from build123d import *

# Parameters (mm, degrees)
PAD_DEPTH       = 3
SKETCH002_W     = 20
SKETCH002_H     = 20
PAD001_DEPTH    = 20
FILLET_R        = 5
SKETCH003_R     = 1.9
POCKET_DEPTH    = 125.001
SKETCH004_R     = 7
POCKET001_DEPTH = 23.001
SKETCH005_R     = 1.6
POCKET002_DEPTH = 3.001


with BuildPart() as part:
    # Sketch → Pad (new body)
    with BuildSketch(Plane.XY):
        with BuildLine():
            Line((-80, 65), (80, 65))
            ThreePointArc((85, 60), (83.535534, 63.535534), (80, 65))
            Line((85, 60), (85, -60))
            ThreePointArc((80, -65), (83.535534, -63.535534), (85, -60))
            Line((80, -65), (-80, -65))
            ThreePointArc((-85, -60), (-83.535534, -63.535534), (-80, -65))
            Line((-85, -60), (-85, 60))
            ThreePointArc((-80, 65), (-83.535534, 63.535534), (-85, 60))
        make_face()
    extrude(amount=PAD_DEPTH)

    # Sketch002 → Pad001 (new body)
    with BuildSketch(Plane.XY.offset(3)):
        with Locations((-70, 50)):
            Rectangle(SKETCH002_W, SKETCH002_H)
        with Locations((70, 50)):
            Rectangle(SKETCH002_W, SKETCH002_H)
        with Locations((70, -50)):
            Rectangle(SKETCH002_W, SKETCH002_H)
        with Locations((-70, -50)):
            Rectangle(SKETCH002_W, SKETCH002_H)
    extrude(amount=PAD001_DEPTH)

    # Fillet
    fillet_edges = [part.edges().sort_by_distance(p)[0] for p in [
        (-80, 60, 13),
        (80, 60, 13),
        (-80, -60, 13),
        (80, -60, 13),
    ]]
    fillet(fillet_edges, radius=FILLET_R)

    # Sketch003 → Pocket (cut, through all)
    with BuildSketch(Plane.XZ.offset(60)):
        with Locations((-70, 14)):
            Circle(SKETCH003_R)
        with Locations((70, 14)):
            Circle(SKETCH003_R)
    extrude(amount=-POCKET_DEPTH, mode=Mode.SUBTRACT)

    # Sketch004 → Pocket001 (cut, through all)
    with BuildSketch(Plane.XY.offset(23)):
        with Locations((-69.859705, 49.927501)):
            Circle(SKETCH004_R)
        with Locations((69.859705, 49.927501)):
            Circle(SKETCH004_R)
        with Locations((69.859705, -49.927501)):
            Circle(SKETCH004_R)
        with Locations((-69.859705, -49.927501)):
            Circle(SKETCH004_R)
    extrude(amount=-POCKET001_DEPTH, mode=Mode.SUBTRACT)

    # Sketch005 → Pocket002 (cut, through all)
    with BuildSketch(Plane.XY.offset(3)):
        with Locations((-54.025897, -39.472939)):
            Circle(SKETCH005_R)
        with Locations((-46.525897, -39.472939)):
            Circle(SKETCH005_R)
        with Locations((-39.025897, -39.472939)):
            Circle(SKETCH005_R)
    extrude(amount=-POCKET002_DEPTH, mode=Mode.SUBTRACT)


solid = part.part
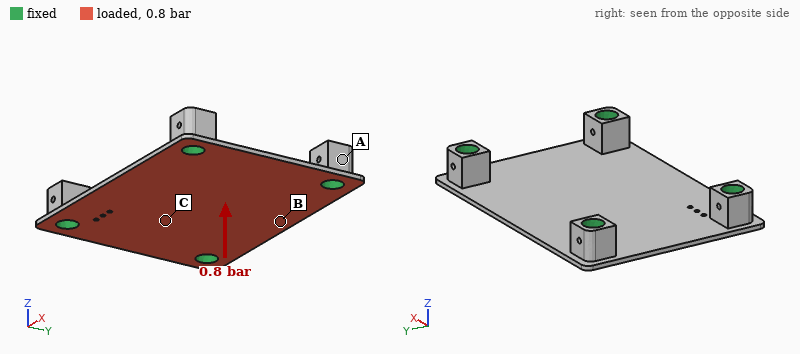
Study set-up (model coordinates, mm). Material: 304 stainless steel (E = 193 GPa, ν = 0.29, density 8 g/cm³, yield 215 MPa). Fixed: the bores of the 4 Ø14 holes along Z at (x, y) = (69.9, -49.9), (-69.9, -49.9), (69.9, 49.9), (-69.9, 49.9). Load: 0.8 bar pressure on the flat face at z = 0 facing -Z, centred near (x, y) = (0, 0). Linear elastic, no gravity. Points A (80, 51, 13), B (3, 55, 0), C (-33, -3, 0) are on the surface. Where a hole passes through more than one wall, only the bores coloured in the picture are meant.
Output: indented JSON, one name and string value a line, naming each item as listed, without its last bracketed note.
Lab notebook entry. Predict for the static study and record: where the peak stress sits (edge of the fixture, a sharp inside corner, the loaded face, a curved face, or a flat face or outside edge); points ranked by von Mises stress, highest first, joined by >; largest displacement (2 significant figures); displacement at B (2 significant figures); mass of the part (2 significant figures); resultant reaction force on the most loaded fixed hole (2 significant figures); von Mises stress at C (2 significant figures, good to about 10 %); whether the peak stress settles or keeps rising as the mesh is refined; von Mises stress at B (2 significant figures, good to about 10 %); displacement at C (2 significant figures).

{
  "where the peak stress sits": "a sharp inside corner",
  "points ranked by von Mises stress, highest first, joined by >": "B > C > A",
  "largest displacement": "0.17 mm",
  "displacement at B": "0.13 mm",
  "mass of the part": "670 g",
  "resultant reaction force on the most loaded fixed hole": "460 N",
  "von Mises stress at C": "20 MPa",
  "whether the peak stress settles or keeps rising as the mesh is refined": "keeps rising",
  "von Mises stress at B": "39 MPa",
  "displacement at C": "0.12 mm"
}
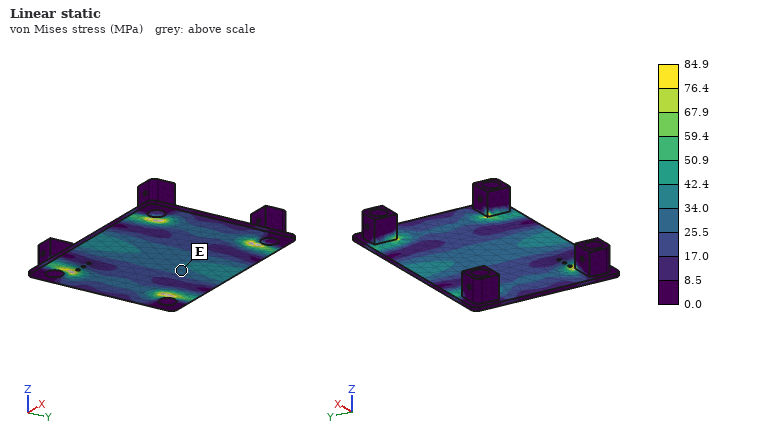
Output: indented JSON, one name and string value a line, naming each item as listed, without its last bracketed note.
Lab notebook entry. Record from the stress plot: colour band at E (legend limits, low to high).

{
  "colour band at E": "25.5 to 34.0 MPa"
}
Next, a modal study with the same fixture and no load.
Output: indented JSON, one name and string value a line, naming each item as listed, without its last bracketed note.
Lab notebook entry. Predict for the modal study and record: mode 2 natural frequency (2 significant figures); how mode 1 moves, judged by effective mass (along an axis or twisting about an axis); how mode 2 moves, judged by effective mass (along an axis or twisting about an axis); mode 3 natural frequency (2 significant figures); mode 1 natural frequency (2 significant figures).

{
  "mode 2 natural frequency": "1200 Hz",
  "how mode 1 moves, judged by effective mass": "along Z",
  "how mode 2 moves, judged by effective mass": "twisting about X",
  "mode 3 natural frequency": "1600 Hz",
  "mode 1 natural frequency": "850 Hz"
}
